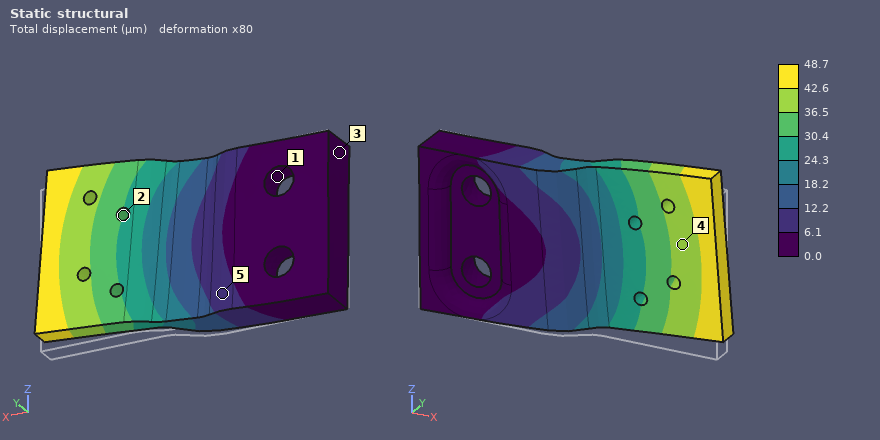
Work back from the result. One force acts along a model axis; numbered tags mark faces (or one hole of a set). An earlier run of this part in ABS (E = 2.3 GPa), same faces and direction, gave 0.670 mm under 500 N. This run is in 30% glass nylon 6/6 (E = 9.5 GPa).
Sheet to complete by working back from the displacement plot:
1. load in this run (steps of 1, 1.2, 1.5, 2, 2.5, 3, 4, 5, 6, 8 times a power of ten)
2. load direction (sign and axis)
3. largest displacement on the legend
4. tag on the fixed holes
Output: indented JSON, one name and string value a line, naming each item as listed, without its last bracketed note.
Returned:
{
  "load in this run": "150 N",
  "load direction": "+Z",
  "largest displacement on the legend": "48.7 µm",
  "tag on the fixed holes": "1"
}
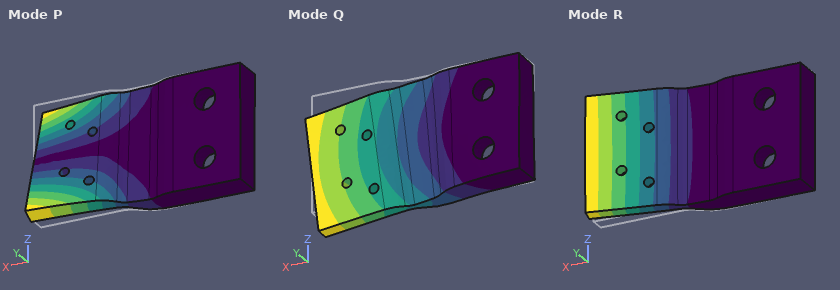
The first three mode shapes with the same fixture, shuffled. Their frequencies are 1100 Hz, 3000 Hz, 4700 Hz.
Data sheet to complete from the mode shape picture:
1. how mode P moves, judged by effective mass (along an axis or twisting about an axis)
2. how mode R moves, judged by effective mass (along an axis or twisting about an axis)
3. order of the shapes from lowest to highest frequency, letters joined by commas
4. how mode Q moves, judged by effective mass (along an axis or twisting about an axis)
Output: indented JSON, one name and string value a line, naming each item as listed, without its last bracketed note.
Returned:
{
  "how mode P moves, judged by effective mass": "twisting about X",
  "how mode R moves, judged by effective mass": "along Y",
  "order of the shapes from lowest to highest frequency, letters joined by commas": "R, P, Q",
  "how mode Q moves, judged by effective mass": "along Z"
}
